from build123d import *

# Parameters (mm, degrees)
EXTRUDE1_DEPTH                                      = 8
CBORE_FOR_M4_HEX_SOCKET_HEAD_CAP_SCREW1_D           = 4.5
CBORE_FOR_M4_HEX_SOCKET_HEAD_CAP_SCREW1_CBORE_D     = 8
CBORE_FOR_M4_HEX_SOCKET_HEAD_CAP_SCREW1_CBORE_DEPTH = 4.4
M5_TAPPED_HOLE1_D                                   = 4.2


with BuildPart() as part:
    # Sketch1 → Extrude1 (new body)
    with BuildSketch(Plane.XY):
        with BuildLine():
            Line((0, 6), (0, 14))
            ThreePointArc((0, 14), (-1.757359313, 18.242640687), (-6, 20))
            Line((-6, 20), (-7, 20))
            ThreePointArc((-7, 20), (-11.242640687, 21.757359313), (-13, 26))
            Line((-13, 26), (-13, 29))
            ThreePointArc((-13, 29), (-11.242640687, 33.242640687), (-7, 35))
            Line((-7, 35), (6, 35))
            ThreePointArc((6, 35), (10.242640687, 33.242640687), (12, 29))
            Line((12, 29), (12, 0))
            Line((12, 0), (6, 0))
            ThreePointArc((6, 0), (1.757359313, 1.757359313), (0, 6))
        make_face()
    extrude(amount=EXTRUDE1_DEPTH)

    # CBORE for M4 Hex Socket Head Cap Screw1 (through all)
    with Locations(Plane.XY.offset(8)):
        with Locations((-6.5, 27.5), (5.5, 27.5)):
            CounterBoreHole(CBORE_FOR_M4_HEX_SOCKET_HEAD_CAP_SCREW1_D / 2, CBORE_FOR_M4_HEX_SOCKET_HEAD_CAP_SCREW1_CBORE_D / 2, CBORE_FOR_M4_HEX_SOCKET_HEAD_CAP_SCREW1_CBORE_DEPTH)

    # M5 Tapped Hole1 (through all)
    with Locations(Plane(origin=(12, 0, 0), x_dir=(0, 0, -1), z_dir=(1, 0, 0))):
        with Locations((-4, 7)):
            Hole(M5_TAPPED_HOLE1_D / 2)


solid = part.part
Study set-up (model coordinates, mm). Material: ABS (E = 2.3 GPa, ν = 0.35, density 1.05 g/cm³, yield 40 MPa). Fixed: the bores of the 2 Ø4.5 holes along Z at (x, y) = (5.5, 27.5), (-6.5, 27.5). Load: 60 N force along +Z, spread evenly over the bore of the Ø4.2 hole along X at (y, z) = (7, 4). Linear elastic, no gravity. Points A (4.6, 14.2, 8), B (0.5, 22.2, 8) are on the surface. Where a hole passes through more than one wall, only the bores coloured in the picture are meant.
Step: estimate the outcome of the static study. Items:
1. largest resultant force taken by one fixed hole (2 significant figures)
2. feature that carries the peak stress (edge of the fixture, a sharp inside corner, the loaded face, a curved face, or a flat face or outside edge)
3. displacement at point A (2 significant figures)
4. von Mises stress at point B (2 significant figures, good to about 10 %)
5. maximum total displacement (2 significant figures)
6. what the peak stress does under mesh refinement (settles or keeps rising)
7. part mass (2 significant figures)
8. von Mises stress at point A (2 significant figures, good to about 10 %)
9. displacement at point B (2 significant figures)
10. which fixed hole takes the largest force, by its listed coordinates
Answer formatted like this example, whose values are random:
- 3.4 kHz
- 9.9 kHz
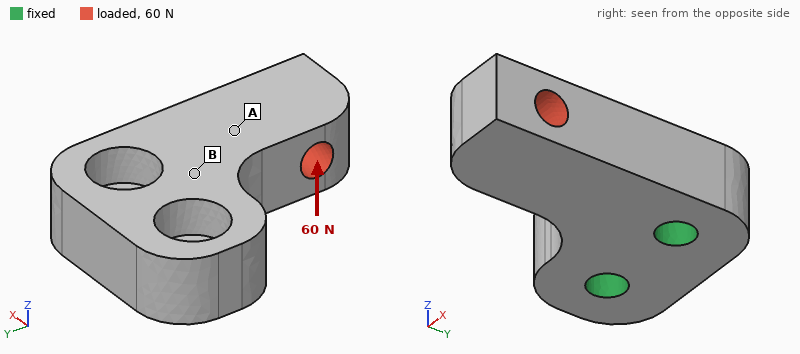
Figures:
- 60 N
- edge of the fixture
- 0.16 mm
- 8.3 MPa
- 0.38 mm
- keeps rising
- 4.2 g
- 3.2 MPa
- 0.061 mm
- (5.5, 27.5)
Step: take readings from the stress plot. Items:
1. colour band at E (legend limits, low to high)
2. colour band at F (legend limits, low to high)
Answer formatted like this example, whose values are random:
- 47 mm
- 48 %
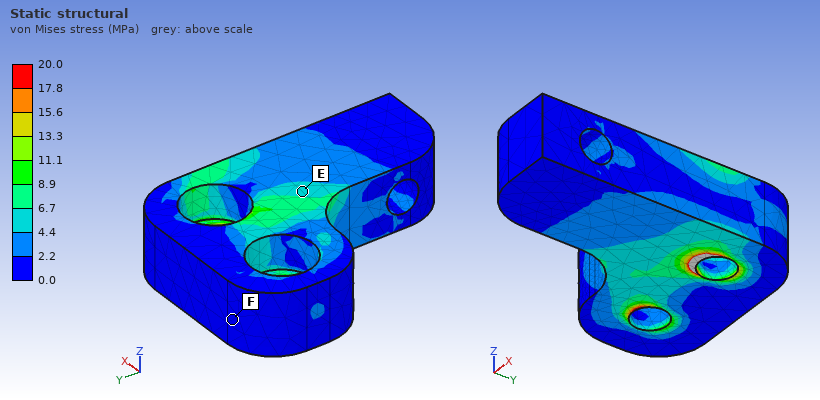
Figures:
- 4.4 to 6.7 MPa
- 0.0 to 2.2 MPa
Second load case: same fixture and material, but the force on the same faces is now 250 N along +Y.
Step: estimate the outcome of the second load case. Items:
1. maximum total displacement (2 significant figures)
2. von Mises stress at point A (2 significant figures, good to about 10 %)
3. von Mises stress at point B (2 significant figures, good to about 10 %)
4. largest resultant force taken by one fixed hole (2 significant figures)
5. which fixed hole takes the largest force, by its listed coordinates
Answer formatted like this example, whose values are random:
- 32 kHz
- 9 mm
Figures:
- 0.14 mm
- 2.6 MPa
- 3.9 MPa
- 230 N
- (5.5, 27.5)
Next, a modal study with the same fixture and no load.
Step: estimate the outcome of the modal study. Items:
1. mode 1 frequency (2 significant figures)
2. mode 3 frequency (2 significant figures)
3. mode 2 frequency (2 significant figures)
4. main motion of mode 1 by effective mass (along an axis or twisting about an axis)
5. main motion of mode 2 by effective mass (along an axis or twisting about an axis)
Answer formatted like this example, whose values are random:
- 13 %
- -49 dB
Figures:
- 2100 Hz
- 8000 Hz
- 4300 Hz
- along Z
- along X
